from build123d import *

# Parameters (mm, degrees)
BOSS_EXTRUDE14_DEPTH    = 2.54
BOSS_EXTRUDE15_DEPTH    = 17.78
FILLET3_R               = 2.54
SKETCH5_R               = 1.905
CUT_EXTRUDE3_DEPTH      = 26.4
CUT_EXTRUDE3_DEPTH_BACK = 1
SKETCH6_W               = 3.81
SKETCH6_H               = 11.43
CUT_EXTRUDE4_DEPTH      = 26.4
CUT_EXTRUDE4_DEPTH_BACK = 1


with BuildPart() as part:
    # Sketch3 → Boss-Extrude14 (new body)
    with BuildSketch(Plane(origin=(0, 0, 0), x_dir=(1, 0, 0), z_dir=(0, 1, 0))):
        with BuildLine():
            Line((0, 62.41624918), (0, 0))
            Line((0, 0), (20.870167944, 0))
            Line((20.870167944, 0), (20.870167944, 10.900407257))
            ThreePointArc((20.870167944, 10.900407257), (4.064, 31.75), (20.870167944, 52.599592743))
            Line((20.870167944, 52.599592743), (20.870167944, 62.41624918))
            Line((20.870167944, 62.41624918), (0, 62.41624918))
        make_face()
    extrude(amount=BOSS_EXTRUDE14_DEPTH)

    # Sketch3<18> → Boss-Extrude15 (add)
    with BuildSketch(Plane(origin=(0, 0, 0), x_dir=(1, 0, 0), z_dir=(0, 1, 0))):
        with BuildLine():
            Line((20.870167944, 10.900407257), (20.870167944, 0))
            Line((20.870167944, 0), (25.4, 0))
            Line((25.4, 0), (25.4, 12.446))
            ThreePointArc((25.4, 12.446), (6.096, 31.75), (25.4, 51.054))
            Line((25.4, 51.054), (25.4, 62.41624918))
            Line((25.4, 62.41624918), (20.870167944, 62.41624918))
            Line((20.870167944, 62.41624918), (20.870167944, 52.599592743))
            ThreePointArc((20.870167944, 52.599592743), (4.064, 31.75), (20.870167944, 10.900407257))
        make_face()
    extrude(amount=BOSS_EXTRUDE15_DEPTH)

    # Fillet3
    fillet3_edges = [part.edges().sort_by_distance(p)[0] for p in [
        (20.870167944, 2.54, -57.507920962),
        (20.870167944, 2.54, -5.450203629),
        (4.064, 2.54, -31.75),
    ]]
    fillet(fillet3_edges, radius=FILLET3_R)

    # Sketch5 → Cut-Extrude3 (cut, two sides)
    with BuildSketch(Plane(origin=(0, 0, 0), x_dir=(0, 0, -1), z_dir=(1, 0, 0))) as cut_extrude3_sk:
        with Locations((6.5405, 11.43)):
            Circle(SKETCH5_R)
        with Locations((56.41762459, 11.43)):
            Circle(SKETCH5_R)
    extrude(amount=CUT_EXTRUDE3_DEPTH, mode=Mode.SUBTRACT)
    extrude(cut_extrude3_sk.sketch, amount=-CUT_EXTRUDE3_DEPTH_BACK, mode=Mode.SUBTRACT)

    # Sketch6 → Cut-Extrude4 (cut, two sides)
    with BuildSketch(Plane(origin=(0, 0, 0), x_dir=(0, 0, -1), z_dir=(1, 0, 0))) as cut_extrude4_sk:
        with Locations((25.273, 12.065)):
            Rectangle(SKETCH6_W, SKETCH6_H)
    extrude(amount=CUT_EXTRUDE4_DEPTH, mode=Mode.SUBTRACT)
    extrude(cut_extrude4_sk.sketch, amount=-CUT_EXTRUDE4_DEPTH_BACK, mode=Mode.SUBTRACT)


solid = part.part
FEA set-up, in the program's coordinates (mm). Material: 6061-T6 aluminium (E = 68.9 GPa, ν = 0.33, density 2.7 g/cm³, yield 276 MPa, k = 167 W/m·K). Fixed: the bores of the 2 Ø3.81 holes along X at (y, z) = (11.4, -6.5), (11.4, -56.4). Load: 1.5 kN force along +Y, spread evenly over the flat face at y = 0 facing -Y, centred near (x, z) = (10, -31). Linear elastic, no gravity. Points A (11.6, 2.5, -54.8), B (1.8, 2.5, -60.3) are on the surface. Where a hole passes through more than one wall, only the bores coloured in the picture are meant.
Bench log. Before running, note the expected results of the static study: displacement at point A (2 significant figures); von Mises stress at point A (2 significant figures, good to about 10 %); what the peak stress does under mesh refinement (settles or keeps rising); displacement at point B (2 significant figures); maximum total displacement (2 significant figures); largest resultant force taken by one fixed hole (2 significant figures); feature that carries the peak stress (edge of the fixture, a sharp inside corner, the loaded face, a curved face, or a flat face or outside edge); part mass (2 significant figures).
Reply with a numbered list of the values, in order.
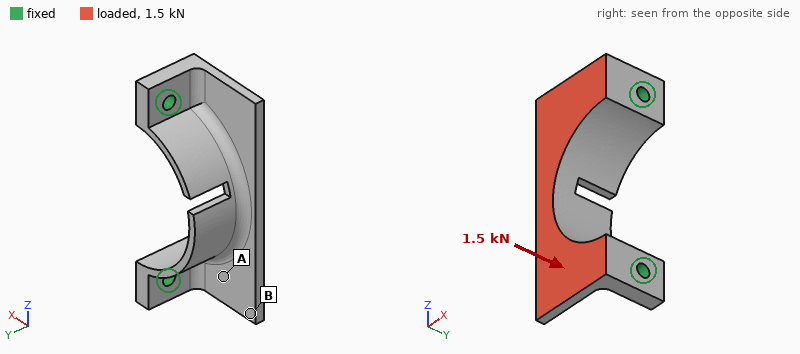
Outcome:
1. 0.084 mm
2. 51 MPa
3. keeps rising
4. 0.21 mm
5. 0.27 mm
6. 760 N
7. edge of the fixture
8. 16 g
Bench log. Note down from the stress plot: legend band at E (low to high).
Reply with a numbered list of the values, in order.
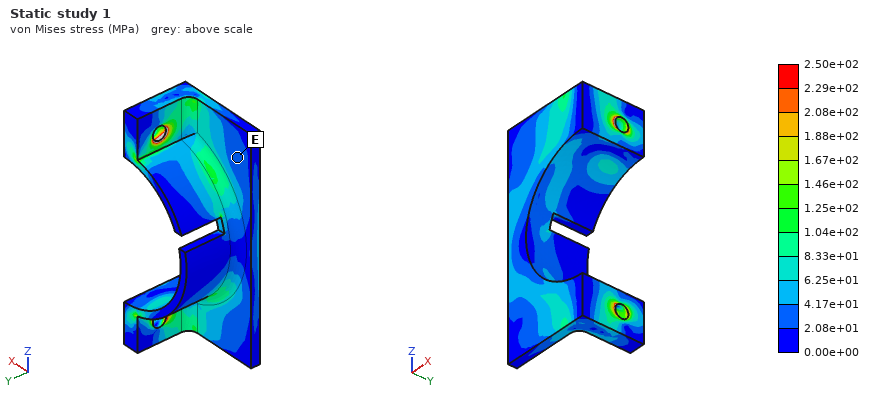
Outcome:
1. 2.08e+01 to 4.17e+01 MPa
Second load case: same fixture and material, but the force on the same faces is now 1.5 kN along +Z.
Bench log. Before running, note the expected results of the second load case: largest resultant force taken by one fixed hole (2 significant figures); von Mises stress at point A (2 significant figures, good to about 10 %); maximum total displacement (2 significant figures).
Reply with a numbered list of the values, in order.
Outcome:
1. 840 N
2. 16 MPa
3. 62 µm
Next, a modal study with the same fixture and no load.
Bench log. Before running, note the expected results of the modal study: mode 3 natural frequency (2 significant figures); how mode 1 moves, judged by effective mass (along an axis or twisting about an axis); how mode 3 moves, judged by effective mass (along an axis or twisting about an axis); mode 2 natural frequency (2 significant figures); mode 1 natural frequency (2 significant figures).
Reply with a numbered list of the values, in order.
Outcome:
1. 8800 Hz
2. along Y
3. along Z
4. 5900 Hz
5. 5400 Hz
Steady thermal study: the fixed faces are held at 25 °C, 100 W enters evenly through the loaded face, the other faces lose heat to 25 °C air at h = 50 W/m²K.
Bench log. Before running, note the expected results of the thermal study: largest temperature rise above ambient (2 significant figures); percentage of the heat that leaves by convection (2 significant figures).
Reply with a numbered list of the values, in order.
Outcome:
1. 79 K
2. 8.9 %
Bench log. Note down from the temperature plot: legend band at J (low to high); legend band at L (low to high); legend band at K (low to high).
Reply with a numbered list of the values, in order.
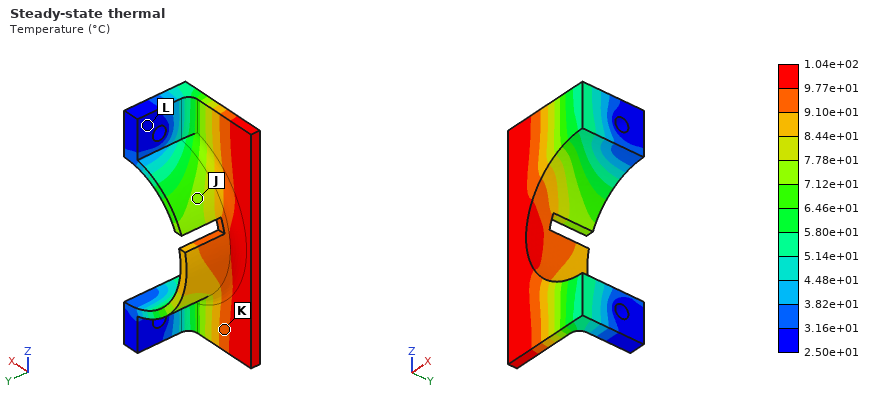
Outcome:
1. 7.12e+01 to 7.78e+01 °C
2. 2.50e+01 to 3.16e+01 °C
3. 9.10e+01 to 9.77e+01 °C
